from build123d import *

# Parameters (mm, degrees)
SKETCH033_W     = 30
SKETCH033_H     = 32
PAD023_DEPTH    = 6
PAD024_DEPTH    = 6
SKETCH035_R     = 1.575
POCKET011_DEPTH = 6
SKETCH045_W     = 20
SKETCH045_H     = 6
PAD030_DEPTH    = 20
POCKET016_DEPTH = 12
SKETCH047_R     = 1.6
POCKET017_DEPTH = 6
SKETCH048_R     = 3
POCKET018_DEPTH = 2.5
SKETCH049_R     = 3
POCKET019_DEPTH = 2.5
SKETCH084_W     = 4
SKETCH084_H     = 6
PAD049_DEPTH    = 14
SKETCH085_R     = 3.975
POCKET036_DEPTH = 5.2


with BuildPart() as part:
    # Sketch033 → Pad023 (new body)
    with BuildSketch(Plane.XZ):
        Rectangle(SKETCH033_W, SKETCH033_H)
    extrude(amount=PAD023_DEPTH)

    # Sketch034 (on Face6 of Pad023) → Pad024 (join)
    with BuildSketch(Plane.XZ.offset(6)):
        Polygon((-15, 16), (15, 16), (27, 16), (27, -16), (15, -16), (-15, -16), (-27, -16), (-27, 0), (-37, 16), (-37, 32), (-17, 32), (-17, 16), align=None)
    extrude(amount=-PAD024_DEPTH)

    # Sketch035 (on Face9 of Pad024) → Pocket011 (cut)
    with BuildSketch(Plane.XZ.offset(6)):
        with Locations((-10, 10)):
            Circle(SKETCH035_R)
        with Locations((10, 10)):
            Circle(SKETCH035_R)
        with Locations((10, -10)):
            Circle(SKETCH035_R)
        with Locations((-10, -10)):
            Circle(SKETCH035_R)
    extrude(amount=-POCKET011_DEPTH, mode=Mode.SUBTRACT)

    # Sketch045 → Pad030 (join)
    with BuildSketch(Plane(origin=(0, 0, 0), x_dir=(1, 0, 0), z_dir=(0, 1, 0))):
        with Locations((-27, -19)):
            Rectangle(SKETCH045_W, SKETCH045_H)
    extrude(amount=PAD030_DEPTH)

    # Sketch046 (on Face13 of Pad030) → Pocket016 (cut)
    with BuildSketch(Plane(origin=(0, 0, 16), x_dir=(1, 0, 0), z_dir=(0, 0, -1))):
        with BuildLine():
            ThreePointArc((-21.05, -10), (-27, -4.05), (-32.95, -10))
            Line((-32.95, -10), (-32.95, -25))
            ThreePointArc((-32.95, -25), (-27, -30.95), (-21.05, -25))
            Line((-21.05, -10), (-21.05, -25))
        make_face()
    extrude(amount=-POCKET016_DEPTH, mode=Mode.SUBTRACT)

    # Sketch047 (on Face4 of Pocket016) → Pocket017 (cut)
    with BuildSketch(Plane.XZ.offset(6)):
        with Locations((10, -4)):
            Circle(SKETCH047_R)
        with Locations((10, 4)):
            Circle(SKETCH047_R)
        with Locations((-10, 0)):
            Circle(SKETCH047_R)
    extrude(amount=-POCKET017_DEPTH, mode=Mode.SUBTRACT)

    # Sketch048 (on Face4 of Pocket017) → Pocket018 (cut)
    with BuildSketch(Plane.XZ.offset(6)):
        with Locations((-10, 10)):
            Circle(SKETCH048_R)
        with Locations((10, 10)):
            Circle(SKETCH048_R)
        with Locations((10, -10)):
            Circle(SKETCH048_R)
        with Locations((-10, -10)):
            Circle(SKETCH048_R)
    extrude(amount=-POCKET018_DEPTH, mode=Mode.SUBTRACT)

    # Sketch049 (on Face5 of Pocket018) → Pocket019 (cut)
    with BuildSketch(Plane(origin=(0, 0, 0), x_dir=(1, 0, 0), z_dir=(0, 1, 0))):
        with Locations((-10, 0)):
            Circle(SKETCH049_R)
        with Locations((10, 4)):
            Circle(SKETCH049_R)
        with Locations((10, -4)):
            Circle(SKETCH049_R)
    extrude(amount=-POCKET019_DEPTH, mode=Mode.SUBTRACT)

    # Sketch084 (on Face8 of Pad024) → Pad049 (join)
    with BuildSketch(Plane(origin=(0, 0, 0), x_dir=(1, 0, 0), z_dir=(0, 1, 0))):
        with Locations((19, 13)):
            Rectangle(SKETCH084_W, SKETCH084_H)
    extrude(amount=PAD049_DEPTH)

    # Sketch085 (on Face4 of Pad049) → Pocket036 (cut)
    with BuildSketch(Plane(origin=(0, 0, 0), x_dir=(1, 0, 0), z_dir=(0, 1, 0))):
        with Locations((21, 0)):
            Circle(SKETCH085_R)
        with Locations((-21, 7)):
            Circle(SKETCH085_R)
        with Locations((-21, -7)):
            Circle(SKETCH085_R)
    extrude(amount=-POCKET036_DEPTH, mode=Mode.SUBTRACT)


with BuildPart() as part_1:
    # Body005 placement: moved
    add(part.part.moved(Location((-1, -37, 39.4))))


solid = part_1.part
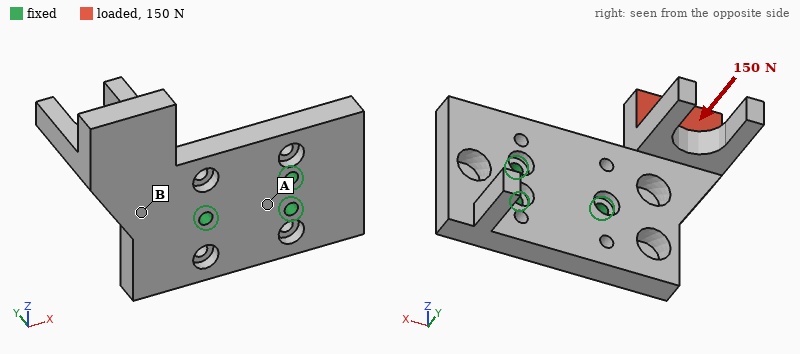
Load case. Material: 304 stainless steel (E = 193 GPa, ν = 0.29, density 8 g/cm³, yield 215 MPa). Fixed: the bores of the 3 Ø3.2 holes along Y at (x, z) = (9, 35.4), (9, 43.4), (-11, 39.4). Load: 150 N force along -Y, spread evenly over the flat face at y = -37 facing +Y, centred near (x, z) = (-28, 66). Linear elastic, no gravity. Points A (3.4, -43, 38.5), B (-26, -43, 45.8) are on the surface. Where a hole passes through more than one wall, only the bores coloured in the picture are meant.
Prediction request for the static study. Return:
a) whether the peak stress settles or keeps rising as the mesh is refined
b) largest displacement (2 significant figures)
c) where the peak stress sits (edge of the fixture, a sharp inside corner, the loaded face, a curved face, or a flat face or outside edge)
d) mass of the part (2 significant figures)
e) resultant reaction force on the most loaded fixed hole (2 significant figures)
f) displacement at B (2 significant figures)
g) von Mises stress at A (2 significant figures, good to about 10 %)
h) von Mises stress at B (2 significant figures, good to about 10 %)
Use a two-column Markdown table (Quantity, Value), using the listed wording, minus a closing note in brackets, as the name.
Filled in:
| Quantity | Value |
|---|---|
| whether the peak stress settles or keeps rising as the mesh is refined | keeps rising |
| largest displacement | 51 µm |
| where the peak stress sits | edge of the fixture |
| mass of the part | 100 g |
| resultant reaction force on the most loaded fixed hole | 270 N |
| displacement at B | 9.7 µm |
| von Mises stress at A | 7.9 MPa |
| von Mises stress at B | 25 MPa |
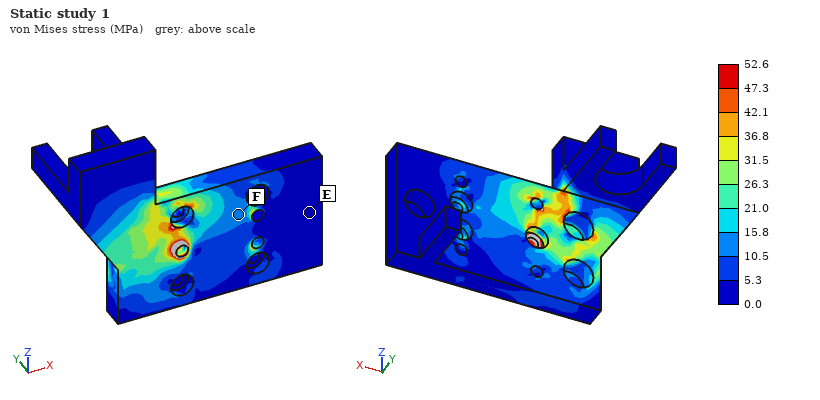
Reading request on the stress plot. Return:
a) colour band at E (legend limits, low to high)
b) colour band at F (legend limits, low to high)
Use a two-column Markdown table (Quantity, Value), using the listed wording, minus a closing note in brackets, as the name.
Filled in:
| Quantity | Value |
|---|---|
| colour band at E | 0.0 to 5.3 MPa |
| colour band at F | 10.5 to 15.8 MPa |
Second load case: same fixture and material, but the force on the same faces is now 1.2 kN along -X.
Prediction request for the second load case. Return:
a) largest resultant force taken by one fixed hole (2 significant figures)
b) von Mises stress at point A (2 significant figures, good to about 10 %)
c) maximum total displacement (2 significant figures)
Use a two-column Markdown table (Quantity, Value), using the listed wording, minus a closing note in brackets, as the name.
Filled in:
| Quantity | Value |
|---|---|
| largest resultant force taken by one fixed hole | 1.3 kN |
| von Mises stress at point A | 12 MPa |
| maximum total displacement | 47 µm |
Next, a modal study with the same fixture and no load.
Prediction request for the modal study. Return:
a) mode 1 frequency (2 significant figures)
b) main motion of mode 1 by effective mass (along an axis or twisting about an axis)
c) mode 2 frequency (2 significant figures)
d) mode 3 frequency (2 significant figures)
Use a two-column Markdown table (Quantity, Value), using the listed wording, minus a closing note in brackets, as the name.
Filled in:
| Quantity | Value |
|---|---|
| mode 1 frequency | 2100 Hz |
| main motion of mode 1 by effective mass | along Y |
| mode 2 frequency | 4700 Hz |
| mode 3 frequency | 7500 Hz |
